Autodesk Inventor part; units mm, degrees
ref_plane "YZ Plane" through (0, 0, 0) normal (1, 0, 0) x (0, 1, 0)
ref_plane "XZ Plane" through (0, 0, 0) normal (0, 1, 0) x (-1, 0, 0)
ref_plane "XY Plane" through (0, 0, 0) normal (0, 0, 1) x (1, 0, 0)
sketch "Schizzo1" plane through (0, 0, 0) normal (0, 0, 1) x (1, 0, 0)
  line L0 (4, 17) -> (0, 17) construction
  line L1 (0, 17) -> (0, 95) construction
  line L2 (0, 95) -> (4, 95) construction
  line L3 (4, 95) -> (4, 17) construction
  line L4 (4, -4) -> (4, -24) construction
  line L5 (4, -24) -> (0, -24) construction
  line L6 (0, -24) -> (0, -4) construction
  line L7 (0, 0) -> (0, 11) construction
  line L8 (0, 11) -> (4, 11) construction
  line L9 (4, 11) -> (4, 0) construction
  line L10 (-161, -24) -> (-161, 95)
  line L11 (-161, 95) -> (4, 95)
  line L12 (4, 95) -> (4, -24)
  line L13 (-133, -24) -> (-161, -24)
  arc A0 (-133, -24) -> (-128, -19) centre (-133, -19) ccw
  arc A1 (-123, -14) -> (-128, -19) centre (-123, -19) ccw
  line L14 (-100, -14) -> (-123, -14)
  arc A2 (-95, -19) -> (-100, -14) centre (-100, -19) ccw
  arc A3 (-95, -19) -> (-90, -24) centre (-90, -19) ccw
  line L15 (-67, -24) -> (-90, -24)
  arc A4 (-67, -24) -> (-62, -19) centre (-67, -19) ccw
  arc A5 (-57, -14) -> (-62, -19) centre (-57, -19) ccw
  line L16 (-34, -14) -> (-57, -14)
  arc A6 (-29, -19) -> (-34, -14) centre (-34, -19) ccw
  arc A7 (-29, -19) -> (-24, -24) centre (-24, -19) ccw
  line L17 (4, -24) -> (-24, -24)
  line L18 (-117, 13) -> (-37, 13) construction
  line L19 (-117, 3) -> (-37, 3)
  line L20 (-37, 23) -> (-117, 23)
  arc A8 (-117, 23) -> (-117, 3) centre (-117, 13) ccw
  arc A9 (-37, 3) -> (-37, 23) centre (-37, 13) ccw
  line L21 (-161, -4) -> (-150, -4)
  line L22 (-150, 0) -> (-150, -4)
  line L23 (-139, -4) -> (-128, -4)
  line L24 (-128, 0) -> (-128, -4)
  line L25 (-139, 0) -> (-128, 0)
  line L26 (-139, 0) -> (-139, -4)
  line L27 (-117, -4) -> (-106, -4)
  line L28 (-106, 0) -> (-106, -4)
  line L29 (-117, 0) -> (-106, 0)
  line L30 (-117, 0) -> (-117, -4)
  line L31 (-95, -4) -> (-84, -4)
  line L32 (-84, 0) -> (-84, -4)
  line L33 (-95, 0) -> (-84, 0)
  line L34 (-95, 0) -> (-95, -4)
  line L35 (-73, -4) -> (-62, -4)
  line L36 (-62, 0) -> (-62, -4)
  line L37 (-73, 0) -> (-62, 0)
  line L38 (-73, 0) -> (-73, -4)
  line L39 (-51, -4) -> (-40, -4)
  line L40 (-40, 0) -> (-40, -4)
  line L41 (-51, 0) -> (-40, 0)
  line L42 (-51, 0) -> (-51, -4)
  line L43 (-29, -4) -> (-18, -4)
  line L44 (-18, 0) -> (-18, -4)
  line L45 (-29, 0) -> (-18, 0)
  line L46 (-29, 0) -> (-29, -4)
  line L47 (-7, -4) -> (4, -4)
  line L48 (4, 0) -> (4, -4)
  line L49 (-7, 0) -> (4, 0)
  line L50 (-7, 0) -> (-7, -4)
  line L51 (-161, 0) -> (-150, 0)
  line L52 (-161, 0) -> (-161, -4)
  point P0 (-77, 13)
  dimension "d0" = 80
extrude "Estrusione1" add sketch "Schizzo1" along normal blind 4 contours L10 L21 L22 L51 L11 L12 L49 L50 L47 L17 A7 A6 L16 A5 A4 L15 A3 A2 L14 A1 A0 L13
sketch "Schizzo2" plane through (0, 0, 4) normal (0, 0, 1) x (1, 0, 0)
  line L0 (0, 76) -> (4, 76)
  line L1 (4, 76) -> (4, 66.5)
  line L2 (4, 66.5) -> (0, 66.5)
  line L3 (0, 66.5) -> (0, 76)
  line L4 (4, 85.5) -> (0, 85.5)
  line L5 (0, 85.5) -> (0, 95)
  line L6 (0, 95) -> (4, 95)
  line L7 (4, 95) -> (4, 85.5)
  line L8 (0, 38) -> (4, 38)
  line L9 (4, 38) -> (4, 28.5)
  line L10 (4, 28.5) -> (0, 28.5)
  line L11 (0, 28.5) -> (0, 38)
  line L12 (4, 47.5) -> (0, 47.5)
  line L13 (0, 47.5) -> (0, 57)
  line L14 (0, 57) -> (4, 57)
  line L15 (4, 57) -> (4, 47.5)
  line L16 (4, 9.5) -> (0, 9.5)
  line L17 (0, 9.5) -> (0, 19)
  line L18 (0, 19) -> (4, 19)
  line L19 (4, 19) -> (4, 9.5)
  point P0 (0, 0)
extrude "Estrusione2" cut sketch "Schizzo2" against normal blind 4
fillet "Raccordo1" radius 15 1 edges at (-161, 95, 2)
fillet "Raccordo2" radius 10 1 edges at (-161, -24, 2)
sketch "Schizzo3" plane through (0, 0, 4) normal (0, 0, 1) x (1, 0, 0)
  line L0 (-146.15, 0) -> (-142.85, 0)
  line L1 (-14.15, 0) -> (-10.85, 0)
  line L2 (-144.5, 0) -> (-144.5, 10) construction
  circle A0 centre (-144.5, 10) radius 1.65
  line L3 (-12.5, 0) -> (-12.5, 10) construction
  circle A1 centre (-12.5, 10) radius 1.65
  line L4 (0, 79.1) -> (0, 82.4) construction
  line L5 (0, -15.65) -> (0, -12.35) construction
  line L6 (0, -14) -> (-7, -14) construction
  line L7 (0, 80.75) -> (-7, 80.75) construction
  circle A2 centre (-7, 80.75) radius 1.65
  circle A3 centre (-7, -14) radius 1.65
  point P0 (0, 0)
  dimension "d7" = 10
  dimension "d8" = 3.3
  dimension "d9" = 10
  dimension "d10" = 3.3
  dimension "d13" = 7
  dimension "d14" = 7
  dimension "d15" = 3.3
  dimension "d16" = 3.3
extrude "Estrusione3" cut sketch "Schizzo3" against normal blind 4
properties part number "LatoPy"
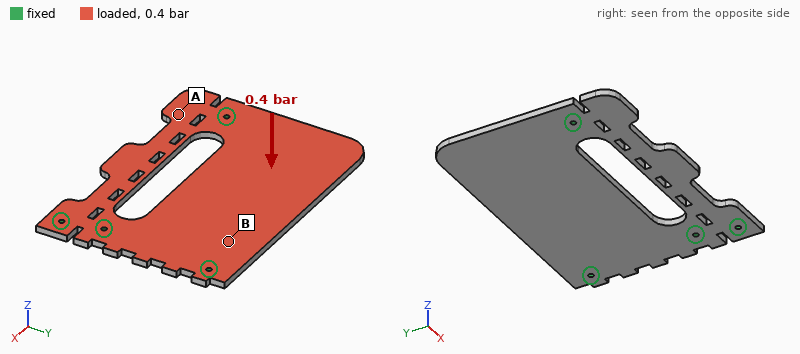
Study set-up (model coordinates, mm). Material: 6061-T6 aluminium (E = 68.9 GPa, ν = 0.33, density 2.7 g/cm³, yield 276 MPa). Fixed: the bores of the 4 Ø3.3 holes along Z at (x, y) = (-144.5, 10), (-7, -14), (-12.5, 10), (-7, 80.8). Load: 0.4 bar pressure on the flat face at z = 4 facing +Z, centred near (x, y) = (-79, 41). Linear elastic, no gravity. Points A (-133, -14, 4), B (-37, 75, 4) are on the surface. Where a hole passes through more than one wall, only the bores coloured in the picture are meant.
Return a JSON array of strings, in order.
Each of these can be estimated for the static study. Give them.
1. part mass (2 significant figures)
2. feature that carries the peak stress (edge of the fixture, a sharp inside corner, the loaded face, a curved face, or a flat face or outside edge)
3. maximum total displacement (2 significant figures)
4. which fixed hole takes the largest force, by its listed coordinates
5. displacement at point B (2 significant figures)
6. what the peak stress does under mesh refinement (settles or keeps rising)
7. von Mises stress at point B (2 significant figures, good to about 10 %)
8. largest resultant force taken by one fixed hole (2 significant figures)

["180 g", "edge of the fixture", "0.74 mm", "(-144.5, 10)", "0.15 mm", "keeps rising", "18 MPa", "300 N"]
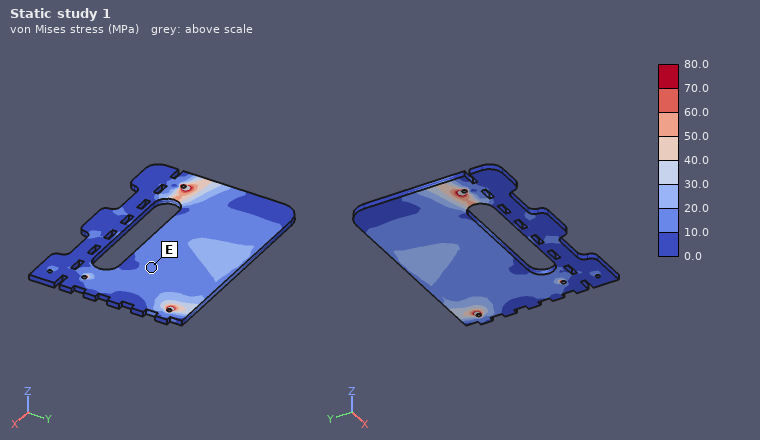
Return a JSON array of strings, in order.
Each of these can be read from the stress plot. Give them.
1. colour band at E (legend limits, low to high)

["10.0 to 20.0 MPa"]
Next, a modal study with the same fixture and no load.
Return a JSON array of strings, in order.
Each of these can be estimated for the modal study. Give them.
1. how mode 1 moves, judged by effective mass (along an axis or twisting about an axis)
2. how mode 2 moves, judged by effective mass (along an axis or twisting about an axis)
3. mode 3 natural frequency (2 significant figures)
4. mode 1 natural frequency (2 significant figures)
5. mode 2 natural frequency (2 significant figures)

["along Z", "along Z", "1100 Hz", "470 Hz", "1000 Hz"]
